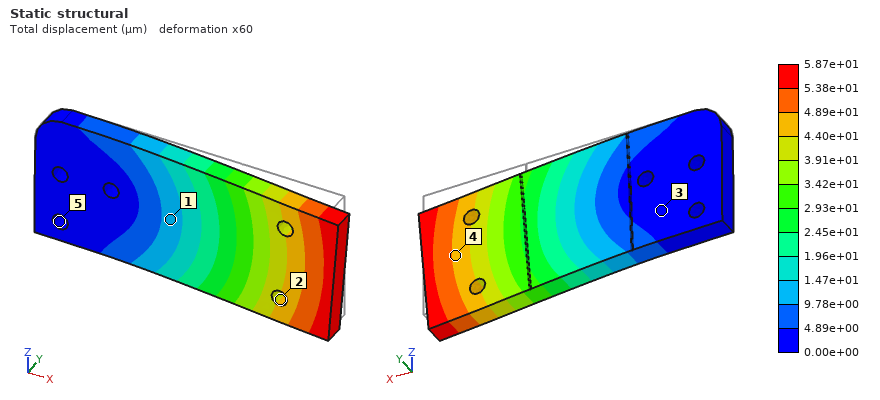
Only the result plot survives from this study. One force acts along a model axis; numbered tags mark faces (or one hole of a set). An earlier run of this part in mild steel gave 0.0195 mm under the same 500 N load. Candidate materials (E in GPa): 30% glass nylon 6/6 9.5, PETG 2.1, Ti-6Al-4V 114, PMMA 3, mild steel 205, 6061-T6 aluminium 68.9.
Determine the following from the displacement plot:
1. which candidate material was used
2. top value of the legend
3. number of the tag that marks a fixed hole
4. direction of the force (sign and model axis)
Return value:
6061-T6 aluminium
5.87e+01 µm
5
-Z
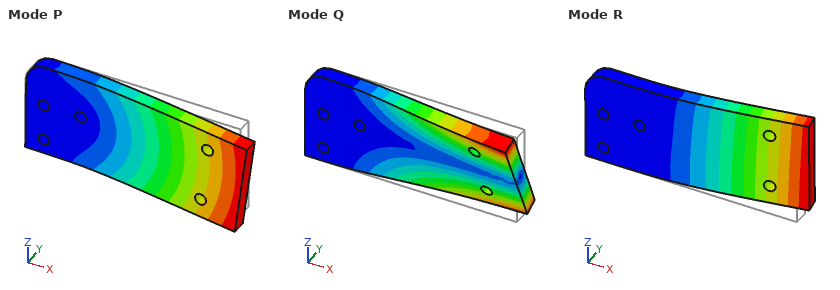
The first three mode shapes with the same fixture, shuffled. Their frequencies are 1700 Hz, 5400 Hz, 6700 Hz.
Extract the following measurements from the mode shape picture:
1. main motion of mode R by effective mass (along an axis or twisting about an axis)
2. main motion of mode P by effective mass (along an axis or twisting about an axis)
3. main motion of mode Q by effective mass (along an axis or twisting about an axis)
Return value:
along Y
along Z
twisting about X
